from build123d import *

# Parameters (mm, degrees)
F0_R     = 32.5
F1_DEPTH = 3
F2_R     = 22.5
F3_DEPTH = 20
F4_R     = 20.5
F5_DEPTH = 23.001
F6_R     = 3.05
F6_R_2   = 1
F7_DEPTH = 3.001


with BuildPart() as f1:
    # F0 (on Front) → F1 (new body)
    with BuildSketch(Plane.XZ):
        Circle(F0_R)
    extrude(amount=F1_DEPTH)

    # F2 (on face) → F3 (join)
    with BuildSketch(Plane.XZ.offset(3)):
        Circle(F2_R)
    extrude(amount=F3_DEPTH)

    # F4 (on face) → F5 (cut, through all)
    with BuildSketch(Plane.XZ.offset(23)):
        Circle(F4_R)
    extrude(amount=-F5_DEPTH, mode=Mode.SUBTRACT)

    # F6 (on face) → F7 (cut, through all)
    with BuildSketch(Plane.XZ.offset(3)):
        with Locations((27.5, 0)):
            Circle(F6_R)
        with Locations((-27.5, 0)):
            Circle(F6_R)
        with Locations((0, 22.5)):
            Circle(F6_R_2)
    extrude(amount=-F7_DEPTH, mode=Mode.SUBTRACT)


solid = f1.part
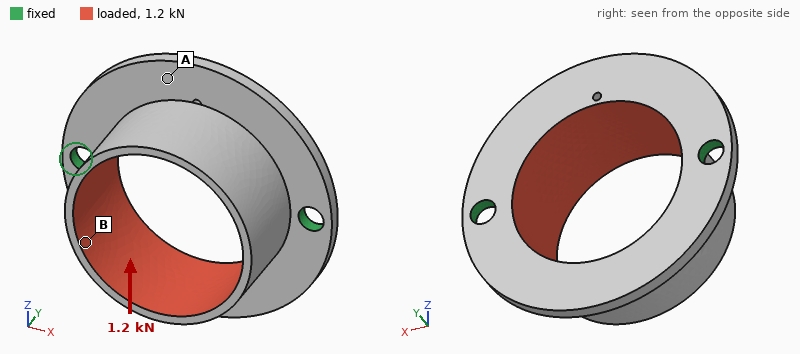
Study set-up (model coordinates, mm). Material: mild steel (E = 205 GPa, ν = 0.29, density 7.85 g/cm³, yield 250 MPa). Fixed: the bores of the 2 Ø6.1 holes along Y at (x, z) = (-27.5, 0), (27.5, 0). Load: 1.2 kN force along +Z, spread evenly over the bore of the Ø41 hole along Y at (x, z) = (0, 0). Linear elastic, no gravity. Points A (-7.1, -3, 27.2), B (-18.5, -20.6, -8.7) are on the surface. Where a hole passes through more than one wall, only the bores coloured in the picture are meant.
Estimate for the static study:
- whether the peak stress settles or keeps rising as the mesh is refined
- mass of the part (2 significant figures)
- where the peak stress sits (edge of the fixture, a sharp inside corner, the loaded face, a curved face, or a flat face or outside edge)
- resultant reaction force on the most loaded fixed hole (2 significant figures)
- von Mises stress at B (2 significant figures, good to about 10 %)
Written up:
keeps rising
88 g
edge of the fixture
600 N
31 MPa
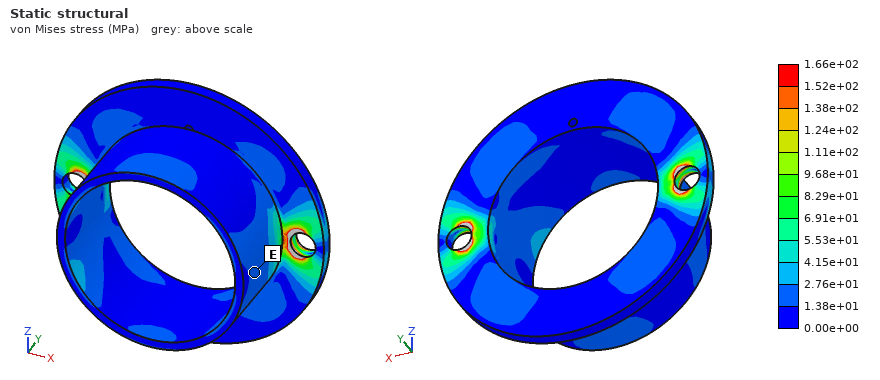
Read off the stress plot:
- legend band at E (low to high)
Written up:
1.38e+01 to 2.76e+01 MPa
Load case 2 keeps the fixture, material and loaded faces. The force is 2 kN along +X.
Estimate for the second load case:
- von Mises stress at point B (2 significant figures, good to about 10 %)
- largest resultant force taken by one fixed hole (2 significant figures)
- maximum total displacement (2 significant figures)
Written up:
10 MPa
1.1 kN
9.0 µm
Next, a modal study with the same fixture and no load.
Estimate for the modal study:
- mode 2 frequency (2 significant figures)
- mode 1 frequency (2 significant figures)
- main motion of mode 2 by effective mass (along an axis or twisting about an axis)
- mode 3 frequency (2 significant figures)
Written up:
3400 Hz
2300 Hz
along Y
5200 Hz
